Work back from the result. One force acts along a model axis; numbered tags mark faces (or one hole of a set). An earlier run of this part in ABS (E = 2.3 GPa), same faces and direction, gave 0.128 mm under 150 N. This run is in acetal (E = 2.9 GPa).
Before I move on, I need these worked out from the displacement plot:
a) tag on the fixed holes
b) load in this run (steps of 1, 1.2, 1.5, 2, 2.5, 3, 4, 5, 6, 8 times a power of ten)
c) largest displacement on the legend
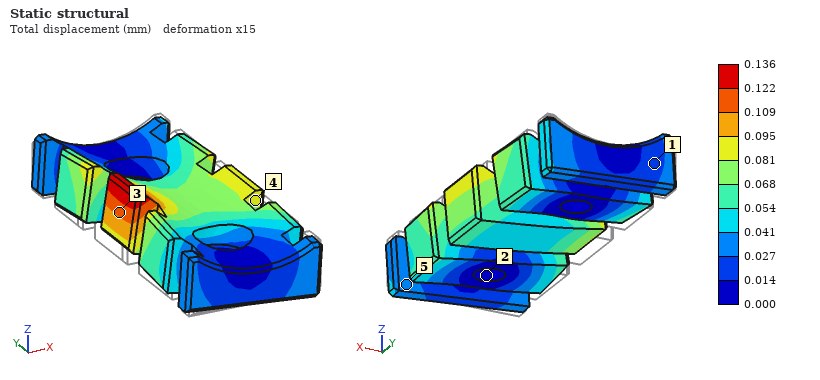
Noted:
2
200 N
0.136 mm
